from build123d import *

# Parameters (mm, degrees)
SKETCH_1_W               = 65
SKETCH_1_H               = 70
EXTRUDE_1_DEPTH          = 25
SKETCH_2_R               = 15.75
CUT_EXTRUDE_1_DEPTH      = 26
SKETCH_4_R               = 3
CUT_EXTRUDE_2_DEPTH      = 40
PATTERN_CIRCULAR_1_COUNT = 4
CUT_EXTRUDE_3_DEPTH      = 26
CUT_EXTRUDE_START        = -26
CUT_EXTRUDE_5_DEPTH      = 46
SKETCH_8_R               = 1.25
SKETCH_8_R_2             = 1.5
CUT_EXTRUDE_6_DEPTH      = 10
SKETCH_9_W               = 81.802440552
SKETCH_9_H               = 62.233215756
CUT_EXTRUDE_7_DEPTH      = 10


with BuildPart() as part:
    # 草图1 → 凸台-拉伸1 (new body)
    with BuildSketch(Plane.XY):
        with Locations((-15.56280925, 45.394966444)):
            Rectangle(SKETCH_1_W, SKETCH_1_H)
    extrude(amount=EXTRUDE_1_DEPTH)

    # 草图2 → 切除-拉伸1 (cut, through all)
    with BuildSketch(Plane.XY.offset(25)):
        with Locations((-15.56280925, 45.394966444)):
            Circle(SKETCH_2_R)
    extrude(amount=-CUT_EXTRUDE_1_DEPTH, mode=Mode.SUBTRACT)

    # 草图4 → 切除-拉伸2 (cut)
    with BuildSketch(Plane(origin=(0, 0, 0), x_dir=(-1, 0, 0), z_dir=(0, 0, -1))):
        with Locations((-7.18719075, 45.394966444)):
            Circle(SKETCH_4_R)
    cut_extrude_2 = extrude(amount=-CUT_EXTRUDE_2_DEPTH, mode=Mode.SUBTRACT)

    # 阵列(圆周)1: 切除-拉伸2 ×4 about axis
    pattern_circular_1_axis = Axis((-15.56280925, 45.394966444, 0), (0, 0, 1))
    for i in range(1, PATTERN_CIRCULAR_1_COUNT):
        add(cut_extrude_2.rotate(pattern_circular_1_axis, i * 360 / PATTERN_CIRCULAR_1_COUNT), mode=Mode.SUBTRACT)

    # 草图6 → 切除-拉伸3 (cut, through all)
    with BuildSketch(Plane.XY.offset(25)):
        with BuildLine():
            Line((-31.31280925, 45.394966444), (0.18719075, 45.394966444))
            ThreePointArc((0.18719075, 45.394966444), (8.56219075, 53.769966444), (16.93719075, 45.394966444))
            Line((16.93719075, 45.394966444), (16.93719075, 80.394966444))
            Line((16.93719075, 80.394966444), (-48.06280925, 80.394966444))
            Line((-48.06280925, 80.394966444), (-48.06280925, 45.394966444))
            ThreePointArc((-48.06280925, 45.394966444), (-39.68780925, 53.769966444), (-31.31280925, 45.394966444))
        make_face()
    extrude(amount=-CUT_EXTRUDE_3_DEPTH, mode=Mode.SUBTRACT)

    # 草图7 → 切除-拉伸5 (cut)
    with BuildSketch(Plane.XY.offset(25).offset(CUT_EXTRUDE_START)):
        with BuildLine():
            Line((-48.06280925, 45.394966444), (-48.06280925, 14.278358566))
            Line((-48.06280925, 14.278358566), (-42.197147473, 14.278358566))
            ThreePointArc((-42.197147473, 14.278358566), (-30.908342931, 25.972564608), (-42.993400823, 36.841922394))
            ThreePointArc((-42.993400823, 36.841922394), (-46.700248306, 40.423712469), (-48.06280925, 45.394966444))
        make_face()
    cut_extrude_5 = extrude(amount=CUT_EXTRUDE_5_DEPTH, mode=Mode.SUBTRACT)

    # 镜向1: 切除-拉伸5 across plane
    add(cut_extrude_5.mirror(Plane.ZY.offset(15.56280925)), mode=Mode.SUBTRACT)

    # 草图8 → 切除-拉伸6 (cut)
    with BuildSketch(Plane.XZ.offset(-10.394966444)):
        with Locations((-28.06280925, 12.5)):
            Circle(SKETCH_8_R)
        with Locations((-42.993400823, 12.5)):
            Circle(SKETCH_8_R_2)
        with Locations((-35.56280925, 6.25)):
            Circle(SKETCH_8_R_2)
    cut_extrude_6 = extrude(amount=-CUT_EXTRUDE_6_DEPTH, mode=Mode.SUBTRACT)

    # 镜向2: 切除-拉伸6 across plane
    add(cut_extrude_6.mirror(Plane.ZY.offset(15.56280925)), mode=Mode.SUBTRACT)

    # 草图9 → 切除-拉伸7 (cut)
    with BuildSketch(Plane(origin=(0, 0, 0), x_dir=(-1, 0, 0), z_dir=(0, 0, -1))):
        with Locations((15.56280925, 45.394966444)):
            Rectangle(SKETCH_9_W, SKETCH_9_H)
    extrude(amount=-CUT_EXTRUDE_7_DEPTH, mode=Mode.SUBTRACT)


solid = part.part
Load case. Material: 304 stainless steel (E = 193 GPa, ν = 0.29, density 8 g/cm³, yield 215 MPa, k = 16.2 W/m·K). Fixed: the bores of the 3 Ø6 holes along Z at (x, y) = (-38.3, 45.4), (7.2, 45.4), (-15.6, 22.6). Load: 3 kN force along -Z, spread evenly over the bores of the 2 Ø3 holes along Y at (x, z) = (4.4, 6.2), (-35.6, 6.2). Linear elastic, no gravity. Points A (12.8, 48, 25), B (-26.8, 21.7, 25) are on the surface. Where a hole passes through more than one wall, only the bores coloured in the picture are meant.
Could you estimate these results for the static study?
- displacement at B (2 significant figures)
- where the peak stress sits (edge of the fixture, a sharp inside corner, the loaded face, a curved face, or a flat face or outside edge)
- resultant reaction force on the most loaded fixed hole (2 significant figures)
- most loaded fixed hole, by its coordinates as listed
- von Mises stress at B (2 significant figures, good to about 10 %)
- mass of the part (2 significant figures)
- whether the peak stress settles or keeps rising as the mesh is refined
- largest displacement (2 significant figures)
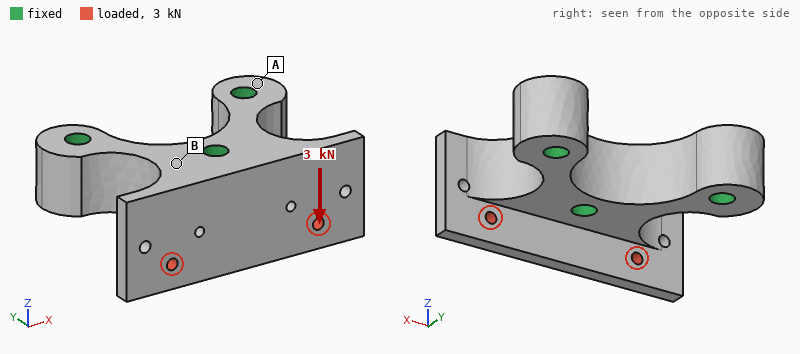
1.9 µm
edge of the fixture
3.0 kN
(-15.6, 22.6)
16 MPa
180 g
keeps rising
11 µm
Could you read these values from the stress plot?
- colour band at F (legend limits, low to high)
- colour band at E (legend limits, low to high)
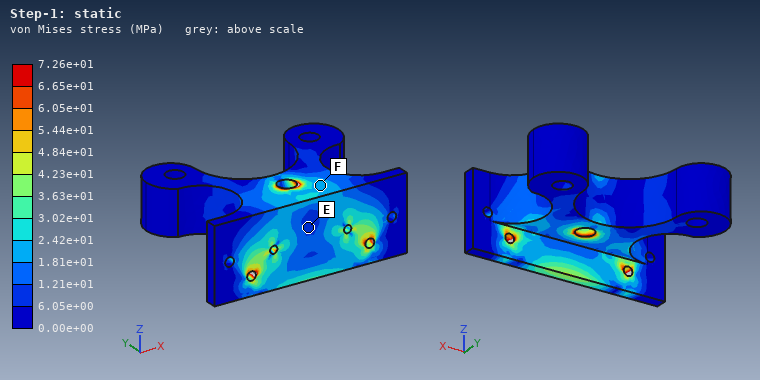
1.81e+01 to 2.42e+01 MPa
6.05e+00 to 1.21e+01 MPa
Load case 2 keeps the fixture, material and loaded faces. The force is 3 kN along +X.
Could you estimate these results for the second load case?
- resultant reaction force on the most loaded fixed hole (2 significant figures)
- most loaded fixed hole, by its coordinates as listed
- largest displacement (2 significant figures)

2.8 kN
(-15.6, 22.6)
14 µm
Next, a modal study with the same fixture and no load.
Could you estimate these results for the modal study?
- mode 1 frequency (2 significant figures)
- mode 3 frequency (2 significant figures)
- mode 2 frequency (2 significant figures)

10000 Hz
12 kHz
11 kHz
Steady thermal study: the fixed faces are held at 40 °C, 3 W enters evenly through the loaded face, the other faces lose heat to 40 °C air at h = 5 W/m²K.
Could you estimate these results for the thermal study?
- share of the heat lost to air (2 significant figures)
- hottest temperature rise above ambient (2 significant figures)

6.2 %
20 K
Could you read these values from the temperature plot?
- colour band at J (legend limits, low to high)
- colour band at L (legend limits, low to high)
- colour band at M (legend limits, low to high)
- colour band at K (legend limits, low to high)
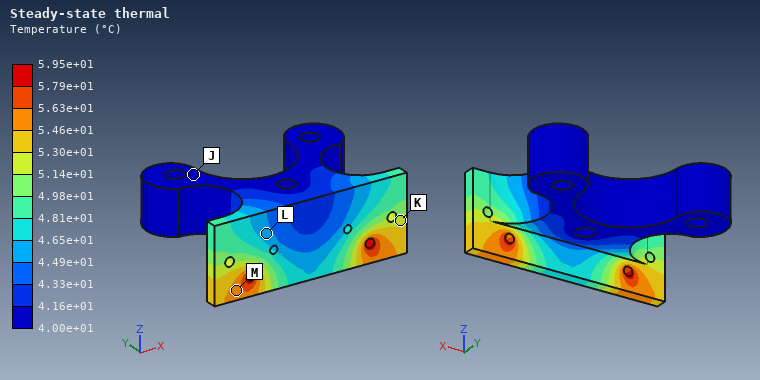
4.00e+01 to 4.16e+01 °C
4.49e+01 to 4.65e+01 °C
5.46e+01 to 5.63e+01 °C
5.14e+01 to 5.30e+01 °C
